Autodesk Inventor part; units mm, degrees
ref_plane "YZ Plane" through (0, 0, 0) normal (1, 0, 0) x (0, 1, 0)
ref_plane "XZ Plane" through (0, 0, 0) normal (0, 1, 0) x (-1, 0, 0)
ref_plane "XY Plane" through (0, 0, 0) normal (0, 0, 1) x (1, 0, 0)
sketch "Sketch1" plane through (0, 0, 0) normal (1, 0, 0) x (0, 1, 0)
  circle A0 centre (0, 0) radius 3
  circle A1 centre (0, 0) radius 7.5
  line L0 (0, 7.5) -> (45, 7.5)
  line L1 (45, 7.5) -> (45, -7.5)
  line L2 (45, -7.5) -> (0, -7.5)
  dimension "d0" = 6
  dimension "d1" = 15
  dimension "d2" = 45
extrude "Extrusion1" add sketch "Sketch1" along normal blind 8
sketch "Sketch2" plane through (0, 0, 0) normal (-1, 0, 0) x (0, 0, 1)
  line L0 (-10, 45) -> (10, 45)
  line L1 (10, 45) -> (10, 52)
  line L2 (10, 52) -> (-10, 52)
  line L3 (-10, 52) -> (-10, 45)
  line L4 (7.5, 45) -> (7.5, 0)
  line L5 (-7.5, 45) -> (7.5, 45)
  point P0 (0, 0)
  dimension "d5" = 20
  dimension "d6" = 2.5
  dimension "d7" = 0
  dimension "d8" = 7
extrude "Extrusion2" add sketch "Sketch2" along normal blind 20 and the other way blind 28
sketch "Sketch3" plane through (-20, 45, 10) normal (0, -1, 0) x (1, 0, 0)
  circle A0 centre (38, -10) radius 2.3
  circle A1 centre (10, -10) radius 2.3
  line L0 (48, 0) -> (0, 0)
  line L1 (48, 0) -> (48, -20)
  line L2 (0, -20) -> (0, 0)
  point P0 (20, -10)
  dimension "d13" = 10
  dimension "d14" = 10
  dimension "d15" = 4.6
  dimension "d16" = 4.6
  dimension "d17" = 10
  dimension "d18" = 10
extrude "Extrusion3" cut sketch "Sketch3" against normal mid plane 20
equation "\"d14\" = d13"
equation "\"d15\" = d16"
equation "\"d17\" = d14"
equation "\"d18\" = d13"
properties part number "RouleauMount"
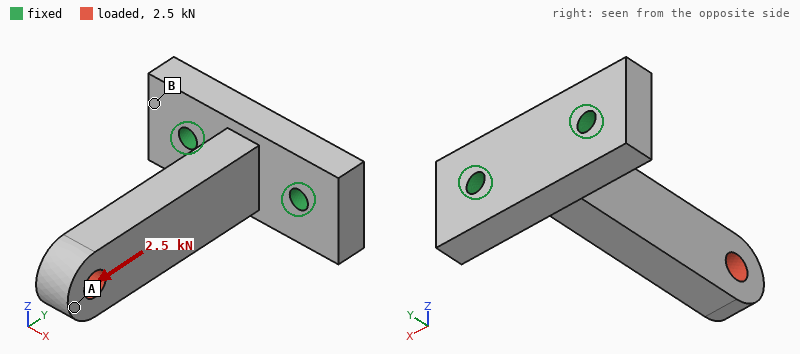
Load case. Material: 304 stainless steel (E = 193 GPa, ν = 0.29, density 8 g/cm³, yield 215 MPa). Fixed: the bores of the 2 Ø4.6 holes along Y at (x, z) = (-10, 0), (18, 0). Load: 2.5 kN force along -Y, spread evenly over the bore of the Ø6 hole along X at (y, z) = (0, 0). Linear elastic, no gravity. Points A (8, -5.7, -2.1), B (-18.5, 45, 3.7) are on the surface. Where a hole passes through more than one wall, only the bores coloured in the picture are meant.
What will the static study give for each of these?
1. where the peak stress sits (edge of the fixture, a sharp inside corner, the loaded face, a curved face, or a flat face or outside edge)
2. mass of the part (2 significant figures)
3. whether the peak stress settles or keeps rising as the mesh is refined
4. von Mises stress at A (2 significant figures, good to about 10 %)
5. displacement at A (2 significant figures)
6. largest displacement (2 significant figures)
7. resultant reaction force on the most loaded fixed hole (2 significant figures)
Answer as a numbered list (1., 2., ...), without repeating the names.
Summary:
1. edge of the fixture
2. 99 g
3. keeps rising
4. 16 MPa
5. 9.3 µm
6. 9.7 µm
7. 1.3 kN
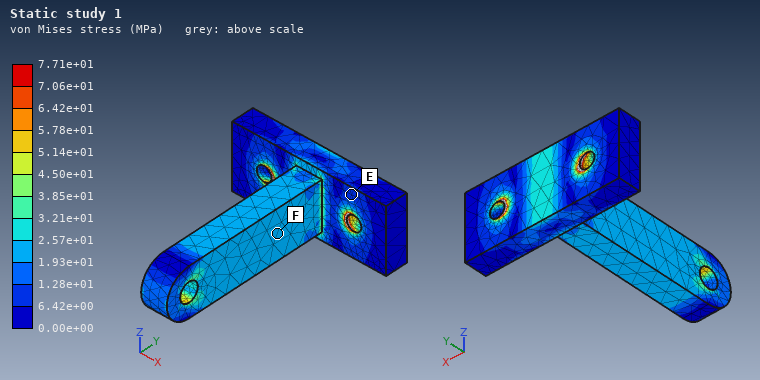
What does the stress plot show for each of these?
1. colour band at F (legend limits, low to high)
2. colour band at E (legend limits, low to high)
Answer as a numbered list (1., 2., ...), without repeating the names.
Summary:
1. 1.93e+01 to 2.57e+01 MPa
2. 6.42e+00 to 1.28e+01 MPa
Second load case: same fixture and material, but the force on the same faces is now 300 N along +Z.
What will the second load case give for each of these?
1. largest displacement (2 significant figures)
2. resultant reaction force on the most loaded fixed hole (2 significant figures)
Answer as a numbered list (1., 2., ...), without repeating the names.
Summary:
1. 60 µm
2. 150 N
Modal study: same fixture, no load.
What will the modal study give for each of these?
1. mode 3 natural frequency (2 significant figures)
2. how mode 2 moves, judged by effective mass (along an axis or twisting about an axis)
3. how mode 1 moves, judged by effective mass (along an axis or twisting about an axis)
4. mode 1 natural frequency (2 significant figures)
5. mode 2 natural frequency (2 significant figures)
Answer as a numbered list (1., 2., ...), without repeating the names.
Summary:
1. 12 kHz
2. along Z
3. along X
4. 2200 Hz
5. 2900 Hz
